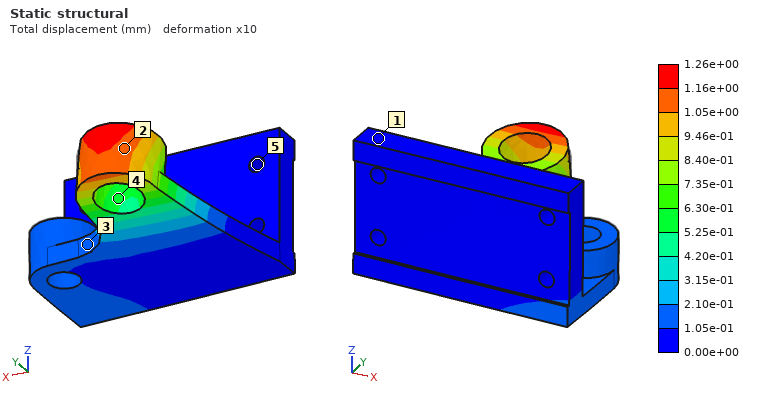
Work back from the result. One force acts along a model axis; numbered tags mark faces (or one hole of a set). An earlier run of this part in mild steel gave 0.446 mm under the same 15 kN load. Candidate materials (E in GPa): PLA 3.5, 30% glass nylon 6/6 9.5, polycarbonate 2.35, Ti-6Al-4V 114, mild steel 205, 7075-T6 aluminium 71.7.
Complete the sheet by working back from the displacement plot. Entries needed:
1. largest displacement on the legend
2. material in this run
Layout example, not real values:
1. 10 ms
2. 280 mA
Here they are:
1. 1.26e+00 mm
2. 7075-T6 aluminium
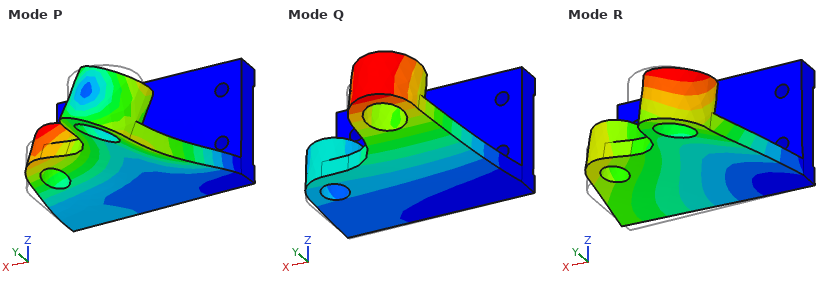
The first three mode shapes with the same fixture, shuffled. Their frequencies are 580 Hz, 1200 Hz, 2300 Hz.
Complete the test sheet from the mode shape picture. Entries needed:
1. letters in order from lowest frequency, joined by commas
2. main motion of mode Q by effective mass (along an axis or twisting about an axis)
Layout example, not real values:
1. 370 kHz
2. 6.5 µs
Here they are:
1. Q, R, P
2. along Z
